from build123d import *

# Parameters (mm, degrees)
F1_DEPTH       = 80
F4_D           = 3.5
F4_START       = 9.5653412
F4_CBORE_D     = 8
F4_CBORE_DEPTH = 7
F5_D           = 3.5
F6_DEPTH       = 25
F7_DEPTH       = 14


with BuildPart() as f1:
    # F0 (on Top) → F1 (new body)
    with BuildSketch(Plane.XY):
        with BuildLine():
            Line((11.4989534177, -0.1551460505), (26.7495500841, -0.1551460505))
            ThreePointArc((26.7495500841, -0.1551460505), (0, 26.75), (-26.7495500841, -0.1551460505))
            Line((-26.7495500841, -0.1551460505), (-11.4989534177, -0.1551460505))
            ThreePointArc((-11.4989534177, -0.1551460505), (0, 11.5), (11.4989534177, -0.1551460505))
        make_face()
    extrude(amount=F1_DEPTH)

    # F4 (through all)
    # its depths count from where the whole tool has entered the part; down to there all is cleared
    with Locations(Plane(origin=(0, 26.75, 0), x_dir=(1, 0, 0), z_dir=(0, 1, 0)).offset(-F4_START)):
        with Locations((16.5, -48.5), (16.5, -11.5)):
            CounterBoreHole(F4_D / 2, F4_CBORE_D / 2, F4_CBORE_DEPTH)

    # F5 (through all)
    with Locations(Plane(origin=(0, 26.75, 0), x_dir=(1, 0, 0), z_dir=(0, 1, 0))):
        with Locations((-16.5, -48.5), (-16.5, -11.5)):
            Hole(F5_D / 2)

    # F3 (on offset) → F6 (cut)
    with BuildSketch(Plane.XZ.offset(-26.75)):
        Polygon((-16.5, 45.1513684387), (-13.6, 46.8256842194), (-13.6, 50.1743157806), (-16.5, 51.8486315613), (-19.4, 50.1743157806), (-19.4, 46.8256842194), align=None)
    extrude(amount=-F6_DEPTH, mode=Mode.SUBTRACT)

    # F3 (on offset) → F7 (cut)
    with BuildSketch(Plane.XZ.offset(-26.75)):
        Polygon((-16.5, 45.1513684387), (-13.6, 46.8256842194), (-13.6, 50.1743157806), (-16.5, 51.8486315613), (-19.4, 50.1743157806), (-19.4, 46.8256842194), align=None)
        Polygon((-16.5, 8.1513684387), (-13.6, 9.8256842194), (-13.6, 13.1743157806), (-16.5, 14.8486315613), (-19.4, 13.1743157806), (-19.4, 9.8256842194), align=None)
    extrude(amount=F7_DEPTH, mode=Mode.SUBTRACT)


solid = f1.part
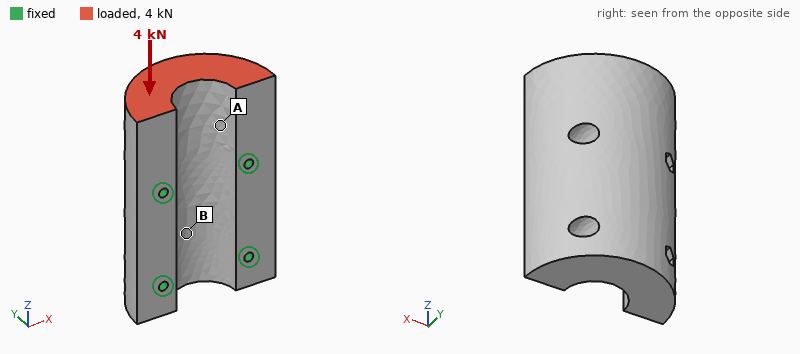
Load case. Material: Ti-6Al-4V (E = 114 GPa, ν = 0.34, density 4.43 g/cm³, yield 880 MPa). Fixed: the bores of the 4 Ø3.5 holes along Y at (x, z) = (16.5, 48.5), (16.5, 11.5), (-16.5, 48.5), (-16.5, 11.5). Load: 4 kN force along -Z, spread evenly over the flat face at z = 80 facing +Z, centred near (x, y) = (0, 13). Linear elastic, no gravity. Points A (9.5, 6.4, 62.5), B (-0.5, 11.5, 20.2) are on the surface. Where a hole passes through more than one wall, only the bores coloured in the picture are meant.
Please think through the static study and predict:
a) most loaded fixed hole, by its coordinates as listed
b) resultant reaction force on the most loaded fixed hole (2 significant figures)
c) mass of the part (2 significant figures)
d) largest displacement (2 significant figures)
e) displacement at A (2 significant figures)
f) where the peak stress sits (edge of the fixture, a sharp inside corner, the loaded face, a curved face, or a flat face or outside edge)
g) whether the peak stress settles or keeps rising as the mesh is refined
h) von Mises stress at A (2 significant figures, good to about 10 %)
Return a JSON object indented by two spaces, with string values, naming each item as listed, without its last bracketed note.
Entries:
{
  "most loaded fixed hole, by its coordinates as listed": "(-16.5, 48.5)",
  "resultant reaction force on the most loaded fixed hole": "1.6 kN",
  "mass of the part": "320 g",
  "largest displacement": "4.0 µm",
  "displacement at A": "1.4 µm",
  "where the peak stress sits": "edge of the fixture",
  "whether the peak stress settles or keeps rising as the mesh is refined": "keeps rising",
  "von Mises stress at A": "5.0 MPa"
}
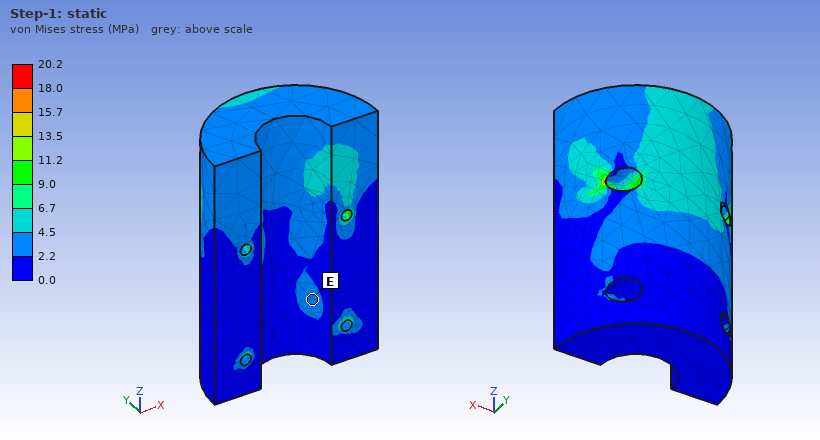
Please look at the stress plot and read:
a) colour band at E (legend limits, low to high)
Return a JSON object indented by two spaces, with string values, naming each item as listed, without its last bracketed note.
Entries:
{
  "colour band at E": "2.2 to 4.5 MPa"
}
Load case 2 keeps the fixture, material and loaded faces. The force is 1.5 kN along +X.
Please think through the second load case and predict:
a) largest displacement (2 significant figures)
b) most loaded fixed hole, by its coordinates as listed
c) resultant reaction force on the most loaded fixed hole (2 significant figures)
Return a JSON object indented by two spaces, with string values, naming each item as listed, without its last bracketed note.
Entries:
{
  "largest displacement": "7.3 µm",
  "most loaded fixed hole, by its coordinates as listed": "(-16.5, 48.5)",
  "resultant reaction force on the most loaded fixed hole": "1.3 kN"
}
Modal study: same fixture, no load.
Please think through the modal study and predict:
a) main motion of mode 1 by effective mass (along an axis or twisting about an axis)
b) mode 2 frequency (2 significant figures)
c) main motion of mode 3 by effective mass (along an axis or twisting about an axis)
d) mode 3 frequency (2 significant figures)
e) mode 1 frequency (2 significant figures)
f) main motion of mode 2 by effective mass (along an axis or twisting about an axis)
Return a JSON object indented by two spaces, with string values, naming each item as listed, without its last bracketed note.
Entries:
{
  "main motion of mode 1 by effective mass": "along Y",
  "mode 2 frequency": "11 kHz",
  "main motion of mode 3 by effective mass": "along X",
  "mode 3 frequency": "16 kHz",
  "mode 1 frequency": "9300 Hz",
  "main motion of mode 2 by effective mass": "along X"
}
